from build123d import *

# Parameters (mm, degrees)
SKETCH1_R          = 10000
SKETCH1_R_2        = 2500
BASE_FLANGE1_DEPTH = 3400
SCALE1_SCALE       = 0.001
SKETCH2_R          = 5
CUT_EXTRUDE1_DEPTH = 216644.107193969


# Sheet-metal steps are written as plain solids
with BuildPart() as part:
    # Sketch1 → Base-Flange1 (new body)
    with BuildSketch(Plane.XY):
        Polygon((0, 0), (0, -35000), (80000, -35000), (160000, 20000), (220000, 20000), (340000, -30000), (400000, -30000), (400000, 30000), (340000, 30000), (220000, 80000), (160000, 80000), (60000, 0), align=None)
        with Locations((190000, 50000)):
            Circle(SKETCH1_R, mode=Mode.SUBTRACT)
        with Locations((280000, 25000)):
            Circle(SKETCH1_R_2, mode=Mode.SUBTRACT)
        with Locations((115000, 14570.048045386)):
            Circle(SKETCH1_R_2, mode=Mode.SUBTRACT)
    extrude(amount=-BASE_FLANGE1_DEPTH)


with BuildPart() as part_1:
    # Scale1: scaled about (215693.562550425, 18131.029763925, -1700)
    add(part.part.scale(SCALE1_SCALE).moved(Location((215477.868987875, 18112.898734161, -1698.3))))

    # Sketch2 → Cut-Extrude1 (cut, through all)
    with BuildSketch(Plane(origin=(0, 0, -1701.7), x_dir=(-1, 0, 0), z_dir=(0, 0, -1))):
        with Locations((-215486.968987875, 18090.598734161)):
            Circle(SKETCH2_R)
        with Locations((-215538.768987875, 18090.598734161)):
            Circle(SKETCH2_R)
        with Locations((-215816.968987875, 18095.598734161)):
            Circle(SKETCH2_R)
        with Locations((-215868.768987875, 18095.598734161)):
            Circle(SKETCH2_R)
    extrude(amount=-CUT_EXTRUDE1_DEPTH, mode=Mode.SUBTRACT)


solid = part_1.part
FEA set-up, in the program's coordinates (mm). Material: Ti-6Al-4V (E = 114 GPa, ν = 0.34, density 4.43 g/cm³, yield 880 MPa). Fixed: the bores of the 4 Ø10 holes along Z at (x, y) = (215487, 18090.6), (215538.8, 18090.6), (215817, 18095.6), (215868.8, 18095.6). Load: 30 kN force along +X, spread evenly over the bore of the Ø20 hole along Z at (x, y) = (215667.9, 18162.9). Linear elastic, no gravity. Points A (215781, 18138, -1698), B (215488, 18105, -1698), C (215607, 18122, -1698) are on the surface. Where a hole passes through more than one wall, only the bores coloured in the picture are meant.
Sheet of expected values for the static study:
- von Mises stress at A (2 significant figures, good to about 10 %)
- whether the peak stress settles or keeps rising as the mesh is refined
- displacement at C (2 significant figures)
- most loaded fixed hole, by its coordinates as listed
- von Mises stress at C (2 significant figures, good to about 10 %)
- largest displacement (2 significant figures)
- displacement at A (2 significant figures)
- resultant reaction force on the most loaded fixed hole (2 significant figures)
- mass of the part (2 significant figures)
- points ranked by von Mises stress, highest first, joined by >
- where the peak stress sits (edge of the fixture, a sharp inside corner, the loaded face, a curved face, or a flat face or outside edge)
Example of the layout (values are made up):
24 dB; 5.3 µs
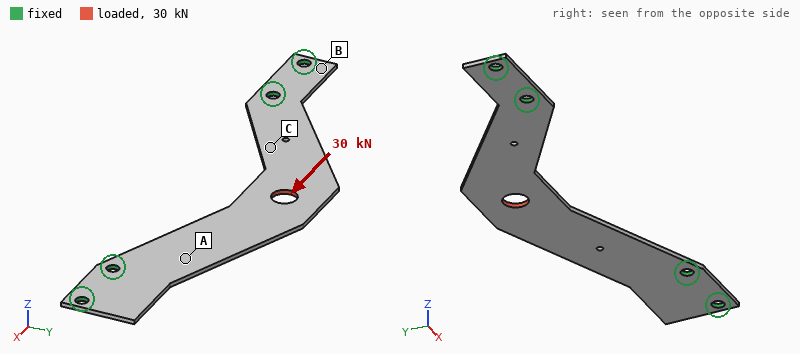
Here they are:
90 MPa; keeps rising; 0.13 mm; (215817, 18095.6); 130 MPa; 0.20 mm; 0.090 mm; 13 kN; 320 g; C > A > B; edge of the fixture
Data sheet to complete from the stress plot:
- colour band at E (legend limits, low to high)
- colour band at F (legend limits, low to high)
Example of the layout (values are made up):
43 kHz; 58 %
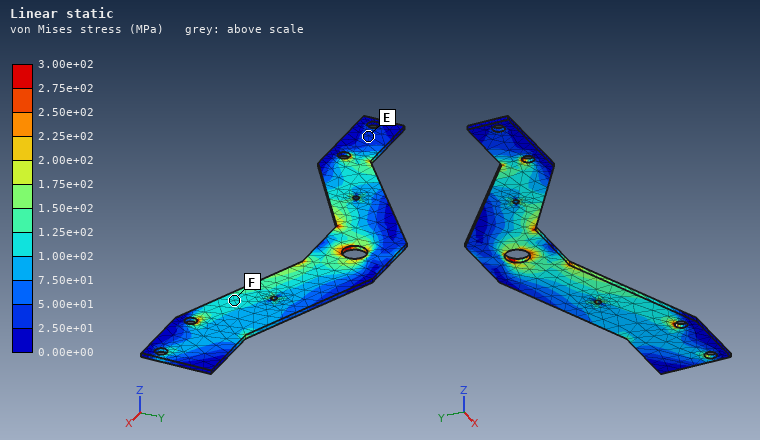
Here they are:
2.50e+01 to 5.00e+01 MPa; 1.00e+02 to 1.25e+02 MPa
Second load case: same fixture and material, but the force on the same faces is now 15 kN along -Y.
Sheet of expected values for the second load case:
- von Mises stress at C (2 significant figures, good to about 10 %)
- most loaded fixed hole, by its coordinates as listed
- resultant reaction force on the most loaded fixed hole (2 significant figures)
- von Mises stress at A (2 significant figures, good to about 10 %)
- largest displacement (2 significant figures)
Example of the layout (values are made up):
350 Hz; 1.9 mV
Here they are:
83 MPa; (215538.8, 18090.6); 13 kN; 55 MPa; 0.27 mm
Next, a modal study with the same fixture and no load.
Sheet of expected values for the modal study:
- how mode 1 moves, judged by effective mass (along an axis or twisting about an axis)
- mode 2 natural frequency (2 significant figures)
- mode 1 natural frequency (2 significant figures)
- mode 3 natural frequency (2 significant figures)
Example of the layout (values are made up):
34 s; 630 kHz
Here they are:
along Z; 460 Hz; 150 Hz; 640 Hz
